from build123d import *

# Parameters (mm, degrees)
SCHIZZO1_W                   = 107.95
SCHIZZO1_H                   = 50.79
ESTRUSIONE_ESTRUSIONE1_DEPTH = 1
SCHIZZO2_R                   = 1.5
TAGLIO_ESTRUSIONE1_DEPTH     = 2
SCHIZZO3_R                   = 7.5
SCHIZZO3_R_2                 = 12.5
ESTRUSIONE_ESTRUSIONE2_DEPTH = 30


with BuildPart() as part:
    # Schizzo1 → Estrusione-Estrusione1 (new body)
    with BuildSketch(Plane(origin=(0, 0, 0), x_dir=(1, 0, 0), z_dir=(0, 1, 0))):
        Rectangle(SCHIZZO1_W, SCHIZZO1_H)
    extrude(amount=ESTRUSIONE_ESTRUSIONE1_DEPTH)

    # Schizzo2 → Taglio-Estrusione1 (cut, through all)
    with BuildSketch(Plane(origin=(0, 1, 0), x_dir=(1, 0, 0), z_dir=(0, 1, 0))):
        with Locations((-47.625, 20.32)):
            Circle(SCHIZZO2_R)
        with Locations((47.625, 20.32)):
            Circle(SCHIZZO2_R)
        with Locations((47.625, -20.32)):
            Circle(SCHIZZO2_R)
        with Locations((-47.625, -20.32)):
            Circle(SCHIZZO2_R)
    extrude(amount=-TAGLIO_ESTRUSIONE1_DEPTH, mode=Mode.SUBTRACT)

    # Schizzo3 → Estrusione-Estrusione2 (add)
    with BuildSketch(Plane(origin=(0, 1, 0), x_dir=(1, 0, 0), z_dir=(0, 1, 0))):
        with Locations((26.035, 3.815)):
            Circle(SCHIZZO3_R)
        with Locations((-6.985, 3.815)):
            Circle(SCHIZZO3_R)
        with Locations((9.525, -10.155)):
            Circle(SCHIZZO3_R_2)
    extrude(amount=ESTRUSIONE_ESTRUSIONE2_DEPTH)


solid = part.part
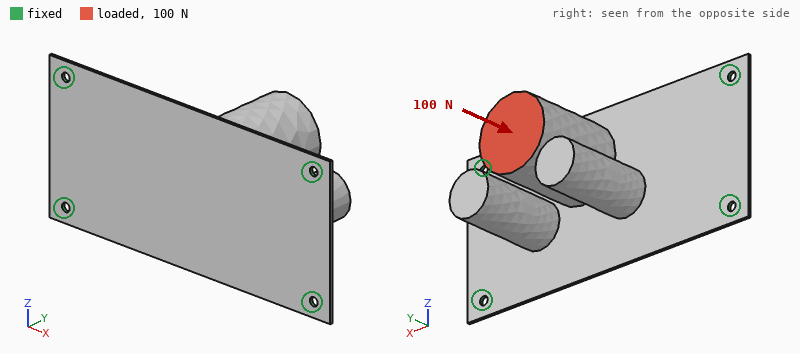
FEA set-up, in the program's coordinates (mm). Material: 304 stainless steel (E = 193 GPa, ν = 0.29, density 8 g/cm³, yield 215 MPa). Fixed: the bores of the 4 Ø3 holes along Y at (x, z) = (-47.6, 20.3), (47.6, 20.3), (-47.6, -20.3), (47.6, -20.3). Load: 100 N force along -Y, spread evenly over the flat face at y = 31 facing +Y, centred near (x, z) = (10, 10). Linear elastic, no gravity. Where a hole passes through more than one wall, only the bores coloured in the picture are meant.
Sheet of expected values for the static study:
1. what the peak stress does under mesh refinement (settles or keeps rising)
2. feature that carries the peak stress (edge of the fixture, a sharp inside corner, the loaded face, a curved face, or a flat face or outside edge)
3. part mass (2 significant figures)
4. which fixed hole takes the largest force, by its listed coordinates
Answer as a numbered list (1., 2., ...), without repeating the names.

1. keeps rising
2. edge of the fixture
3. 250 g
4. (47.6, 20.3)
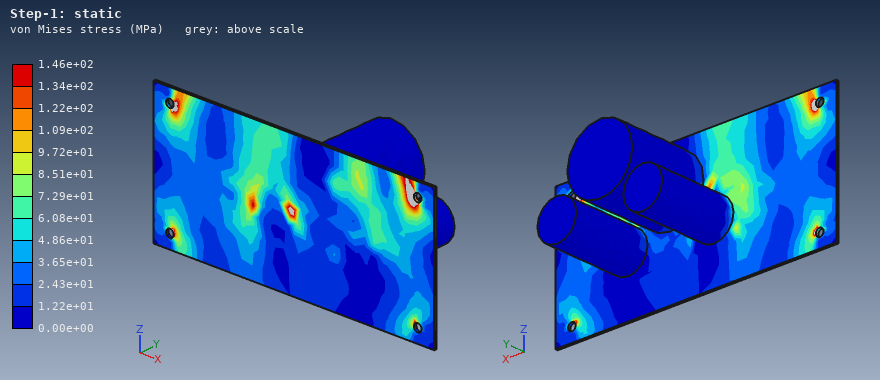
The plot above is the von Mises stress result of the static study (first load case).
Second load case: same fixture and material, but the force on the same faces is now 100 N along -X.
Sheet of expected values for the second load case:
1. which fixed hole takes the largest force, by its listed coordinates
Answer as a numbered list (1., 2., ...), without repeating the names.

1. (-47.6, -20.3)
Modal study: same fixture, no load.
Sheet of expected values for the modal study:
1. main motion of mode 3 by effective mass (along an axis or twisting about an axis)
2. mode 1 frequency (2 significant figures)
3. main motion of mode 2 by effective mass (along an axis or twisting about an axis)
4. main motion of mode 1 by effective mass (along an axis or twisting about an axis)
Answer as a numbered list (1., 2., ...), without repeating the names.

1. along X
2. 220 Hz
3. along Z
4. along Y
